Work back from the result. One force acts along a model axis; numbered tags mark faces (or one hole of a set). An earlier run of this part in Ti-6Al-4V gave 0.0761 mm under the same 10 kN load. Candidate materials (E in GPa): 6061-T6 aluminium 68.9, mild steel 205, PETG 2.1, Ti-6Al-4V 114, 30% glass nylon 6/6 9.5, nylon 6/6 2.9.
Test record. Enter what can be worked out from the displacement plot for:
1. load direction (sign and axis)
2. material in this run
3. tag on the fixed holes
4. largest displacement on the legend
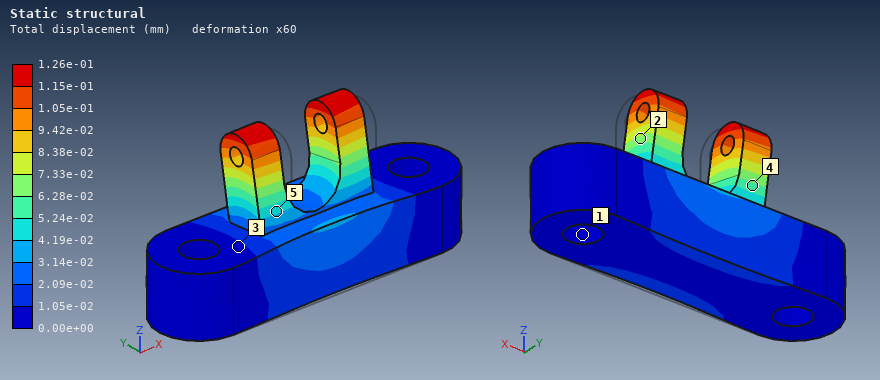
+Y
6061-T6 aluminium
1
1.26e-01 mm
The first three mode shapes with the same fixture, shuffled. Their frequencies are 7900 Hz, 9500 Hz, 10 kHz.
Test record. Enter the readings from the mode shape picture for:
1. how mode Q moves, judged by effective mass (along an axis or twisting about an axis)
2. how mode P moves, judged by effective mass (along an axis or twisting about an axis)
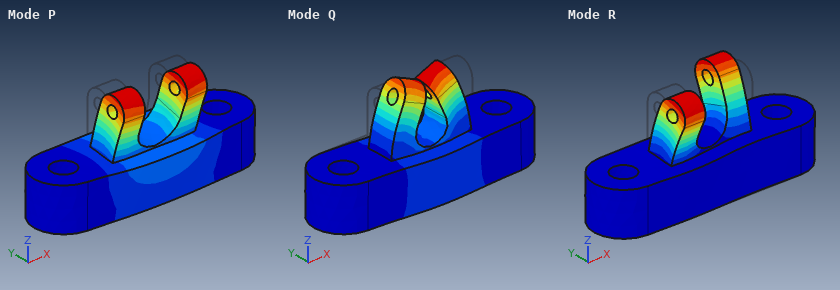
along Z
along Y
